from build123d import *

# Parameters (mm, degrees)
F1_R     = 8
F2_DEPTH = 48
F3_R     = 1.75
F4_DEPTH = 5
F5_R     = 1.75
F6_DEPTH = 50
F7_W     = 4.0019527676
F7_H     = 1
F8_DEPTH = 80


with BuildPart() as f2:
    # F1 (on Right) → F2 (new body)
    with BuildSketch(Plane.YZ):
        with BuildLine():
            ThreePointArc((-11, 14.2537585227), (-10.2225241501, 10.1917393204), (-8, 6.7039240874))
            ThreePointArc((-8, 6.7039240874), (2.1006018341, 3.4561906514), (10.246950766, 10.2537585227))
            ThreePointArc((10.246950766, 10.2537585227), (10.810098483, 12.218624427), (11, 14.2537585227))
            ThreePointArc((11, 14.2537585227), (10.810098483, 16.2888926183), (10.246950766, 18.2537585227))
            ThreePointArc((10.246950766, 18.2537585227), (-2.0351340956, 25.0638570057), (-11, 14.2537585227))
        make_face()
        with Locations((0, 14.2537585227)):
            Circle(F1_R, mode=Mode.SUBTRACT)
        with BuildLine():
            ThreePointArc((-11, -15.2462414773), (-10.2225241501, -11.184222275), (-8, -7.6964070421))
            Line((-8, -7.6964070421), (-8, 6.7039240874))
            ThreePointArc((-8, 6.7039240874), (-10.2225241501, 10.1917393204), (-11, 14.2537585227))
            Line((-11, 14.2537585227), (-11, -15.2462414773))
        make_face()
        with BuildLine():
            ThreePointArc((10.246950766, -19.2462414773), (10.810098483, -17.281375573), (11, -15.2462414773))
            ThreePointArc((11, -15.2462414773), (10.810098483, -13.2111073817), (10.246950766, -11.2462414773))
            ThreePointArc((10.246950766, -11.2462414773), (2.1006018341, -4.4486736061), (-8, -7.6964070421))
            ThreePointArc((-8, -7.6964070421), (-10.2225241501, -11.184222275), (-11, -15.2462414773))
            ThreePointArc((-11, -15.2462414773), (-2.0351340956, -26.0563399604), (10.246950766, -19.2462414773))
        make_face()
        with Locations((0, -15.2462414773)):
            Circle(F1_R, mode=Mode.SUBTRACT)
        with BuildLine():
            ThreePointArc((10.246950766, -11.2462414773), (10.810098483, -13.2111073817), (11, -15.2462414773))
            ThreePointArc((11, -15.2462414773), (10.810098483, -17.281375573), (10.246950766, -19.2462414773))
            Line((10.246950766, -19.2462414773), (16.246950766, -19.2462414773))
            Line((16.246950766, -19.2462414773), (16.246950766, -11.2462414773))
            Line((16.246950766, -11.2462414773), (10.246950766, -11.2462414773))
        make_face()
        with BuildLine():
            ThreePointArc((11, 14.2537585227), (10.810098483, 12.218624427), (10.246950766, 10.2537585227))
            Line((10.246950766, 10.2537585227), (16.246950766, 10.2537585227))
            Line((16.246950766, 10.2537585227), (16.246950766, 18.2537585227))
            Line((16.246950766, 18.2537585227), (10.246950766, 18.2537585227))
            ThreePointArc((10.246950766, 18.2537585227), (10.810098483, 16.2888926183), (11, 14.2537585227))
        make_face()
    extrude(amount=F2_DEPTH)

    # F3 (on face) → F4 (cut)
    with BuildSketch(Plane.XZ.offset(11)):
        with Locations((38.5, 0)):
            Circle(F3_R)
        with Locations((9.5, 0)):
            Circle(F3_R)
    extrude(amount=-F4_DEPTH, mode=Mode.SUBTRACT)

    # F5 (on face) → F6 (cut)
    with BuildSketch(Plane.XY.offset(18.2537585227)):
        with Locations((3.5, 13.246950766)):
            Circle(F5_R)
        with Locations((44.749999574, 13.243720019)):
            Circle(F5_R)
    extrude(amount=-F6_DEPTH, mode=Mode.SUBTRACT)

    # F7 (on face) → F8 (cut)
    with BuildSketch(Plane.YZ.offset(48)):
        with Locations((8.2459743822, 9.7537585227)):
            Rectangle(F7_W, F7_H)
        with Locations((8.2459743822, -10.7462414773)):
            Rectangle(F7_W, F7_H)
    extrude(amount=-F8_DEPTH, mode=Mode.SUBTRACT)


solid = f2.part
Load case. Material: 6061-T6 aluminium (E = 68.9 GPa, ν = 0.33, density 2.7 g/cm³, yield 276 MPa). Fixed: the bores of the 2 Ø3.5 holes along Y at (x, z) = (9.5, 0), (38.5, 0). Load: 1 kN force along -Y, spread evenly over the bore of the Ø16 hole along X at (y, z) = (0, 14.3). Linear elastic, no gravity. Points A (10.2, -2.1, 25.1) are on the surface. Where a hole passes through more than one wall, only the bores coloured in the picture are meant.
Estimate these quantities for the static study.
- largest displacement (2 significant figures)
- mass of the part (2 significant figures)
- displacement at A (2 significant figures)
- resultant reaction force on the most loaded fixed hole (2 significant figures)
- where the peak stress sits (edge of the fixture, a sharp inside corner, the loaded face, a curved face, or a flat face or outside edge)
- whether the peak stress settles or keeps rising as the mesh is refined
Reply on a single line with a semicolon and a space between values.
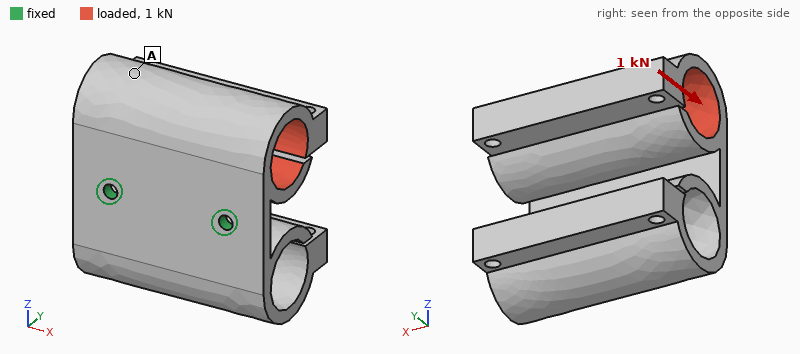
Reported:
0.37 mm; 63 g; 0.30 mm; 500 N; edge of the fixture; keeps rising
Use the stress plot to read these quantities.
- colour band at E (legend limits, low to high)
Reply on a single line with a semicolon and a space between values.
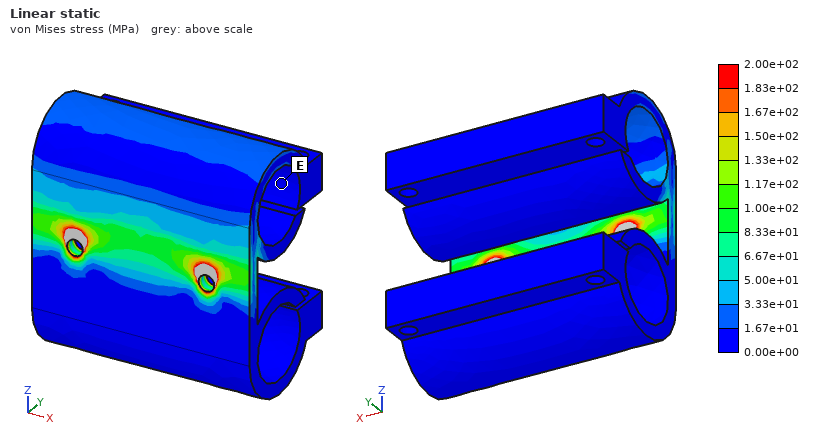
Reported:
0.00e+00 to 1.67e+01 MPa
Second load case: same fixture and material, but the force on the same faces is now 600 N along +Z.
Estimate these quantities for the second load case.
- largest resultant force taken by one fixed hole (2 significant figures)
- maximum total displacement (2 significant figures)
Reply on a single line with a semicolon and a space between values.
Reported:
300 N; 0.33 mm
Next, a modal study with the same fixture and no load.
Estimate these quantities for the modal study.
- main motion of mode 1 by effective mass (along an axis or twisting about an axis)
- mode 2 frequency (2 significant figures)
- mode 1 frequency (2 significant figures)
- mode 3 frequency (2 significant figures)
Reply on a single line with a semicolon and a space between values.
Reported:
along Z; 1200 Hz; 1100 Hz; 1900 Hz
